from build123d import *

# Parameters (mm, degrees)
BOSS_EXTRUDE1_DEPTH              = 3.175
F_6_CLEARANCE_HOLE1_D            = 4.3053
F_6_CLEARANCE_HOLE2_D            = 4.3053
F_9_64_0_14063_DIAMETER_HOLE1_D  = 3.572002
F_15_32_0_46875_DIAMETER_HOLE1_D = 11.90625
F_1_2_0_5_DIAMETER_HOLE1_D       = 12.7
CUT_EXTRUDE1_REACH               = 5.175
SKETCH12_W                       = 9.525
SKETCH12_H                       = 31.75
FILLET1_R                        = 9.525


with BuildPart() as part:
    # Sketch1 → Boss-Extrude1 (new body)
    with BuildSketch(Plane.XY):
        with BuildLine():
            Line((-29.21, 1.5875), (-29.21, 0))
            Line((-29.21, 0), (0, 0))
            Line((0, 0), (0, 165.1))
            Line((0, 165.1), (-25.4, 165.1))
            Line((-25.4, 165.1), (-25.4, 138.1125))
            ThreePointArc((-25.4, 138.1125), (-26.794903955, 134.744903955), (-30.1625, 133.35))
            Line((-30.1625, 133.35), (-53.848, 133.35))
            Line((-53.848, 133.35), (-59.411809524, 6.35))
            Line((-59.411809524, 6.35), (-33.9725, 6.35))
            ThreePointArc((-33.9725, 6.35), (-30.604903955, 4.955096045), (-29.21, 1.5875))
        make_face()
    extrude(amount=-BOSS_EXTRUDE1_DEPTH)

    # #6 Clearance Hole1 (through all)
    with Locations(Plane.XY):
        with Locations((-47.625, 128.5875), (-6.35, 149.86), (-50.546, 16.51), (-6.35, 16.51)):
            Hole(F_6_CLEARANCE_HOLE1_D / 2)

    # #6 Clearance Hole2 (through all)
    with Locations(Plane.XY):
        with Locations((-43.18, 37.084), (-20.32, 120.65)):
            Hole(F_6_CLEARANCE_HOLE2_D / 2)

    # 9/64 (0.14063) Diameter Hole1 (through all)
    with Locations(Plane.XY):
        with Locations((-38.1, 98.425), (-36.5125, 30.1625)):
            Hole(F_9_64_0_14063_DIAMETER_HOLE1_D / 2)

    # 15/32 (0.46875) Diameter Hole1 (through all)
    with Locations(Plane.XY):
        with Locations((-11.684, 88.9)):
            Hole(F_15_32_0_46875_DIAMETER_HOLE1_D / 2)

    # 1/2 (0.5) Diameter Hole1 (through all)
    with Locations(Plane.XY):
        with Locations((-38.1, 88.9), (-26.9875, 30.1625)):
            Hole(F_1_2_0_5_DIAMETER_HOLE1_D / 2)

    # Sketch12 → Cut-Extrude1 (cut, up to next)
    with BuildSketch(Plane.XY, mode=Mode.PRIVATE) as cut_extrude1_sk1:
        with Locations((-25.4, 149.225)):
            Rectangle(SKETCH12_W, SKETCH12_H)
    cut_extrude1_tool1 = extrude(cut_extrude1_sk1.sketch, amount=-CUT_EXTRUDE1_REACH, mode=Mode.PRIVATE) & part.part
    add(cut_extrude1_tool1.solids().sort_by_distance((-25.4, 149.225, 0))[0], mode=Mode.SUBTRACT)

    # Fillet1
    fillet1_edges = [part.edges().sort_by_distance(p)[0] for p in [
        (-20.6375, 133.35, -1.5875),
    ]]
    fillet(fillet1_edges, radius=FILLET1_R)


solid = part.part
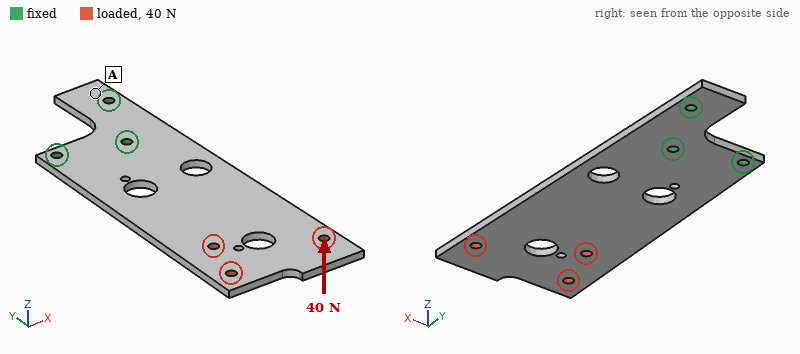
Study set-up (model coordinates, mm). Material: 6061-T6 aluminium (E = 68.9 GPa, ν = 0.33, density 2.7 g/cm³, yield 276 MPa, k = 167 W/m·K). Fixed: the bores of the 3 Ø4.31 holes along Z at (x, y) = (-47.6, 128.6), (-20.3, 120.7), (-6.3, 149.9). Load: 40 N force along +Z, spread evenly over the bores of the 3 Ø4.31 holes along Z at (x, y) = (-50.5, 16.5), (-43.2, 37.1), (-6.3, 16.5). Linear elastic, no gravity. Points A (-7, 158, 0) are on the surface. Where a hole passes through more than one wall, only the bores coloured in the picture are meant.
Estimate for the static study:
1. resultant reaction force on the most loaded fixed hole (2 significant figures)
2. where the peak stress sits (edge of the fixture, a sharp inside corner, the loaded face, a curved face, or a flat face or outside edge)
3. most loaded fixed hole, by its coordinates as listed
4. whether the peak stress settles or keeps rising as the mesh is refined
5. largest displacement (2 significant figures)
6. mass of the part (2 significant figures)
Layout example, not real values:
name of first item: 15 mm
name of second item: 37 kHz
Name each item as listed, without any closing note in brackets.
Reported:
resultant reaction force on the most loaded fixed hole: 90 N
where the peak stress sits: edge of the fixture
most loaded fixed hole, by its coordinates as listed: (-20.3, 120.7)
whether the peak stress settles or keeps rising as the mesh is refined: keeps rising
largest displacement: 1.9 mm
mass of the part: 65 g
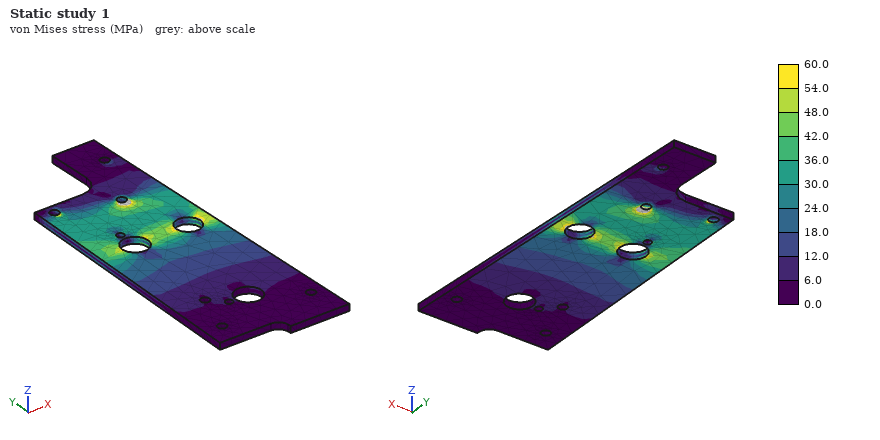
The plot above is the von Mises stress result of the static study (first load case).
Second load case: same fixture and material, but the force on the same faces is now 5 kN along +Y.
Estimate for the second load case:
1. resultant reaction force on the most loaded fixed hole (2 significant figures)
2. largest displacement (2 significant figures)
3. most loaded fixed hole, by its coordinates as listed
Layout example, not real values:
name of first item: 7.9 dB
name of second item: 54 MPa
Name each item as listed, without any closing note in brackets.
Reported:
resultant reaction force on the most loaded fixed hole: 2.5 kN
largest displacement: 0.11 mm
most loaded fixed hole, by its coordinates as listed: (-47.6, 128.6)
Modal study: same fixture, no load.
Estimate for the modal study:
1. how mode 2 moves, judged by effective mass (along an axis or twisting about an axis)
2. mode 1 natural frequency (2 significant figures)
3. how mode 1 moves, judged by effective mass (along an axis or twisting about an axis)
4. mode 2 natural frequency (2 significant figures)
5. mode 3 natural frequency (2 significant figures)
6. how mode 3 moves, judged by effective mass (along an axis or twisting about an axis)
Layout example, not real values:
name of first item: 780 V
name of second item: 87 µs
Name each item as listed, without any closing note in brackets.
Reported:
how mode 2 moves, judged by effective mass: twisting about Y
mode 1 natural frequency: 170 Hz
how mode 1 moves, judged by effective mass: along Z
mode 2 natural frequency: 710 Hz
mode 3 natural frequency: 1100 Hz
how mode 3 moves, judged by effective mass: along Z
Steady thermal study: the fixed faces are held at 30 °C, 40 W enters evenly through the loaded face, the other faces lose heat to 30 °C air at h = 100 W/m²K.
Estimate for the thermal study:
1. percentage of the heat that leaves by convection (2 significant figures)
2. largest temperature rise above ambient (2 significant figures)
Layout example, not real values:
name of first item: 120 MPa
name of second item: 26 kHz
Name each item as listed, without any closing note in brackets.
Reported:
percentage of the heat that leaves by convection: 84 %
largest temperature rise above ambient: 55 K
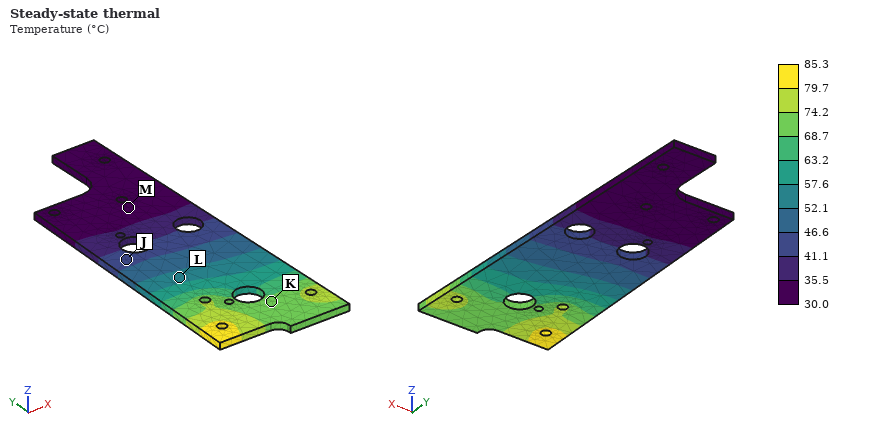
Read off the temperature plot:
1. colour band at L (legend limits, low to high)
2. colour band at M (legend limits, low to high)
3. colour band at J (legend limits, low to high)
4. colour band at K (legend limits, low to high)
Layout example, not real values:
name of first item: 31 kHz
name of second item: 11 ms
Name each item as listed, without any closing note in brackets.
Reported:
colour band at L: 52.1 to 57.6 °C
colour band at M: 30.0 to 35.5 °C
colour band at J: 41.1 to 46.6 °C
colour band at K: 68.7 to 74.2 °C
